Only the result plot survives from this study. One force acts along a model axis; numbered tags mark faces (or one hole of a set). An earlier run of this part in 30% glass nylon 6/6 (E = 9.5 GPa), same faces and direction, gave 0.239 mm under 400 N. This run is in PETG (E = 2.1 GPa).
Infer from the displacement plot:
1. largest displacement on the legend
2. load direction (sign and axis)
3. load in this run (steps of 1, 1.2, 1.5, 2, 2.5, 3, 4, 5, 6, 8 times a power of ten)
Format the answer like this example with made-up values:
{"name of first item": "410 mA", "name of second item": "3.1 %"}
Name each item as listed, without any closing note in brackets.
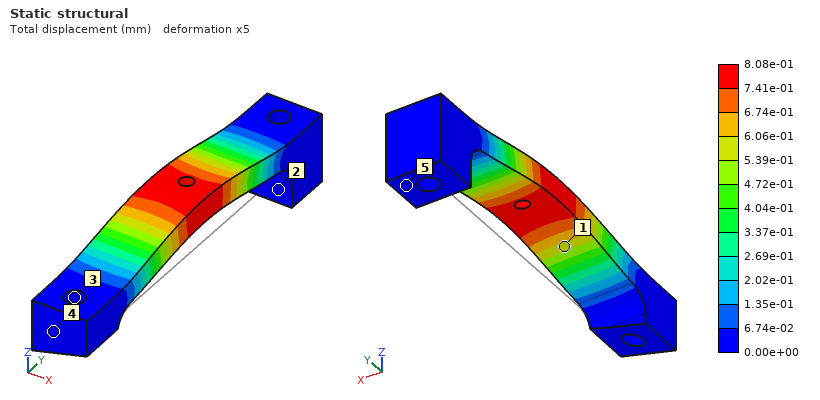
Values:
{"largest displacement on the legend": "8.08e-01 mm", "load direction": "+Z", "load in this run": "300 N"}
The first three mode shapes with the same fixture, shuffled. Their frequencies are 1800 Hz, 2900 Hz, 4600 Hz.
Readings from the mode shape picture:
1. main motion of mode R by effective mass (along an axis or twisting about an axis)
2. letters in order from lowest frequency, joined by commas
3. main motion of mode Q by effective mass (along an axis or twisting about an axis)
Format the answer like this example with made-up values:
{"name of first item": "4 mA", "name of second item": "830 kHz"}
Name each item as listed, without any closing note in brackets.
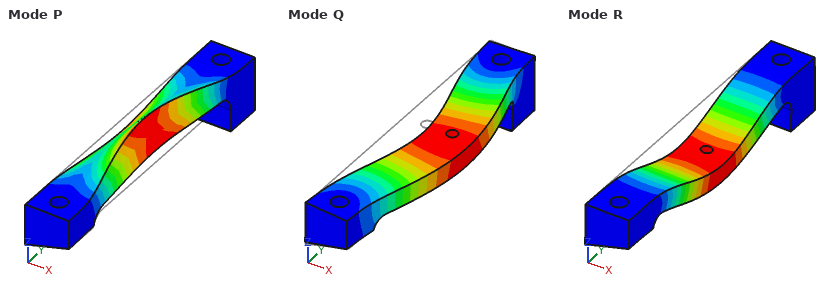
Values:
{"main motion of mode R by effective mass": "along Z", "letters in order from lowest frequency, joined by commas": "R, Q, P", "main motion of mode Q by effective mass": "along X"}
